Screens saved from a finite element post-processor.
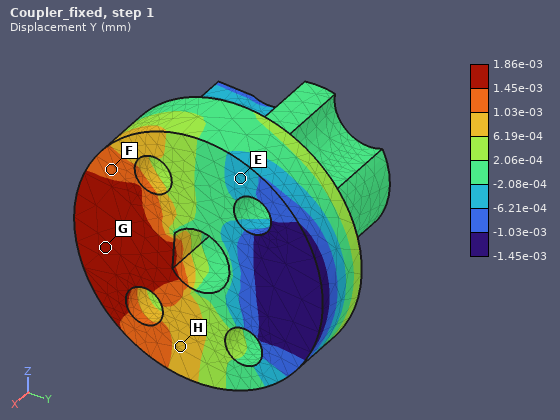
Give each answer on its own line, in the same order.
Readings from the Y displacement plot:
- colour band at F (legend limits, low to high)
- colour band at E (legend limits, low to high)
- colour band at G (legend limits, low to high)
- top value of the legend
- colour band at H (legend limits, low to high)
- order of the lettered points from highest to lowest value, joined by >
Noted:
1.03e-03 to 1.45e-03 mm
-6.21e-04 to -2.08e-04 mm
1.45e-03 to 1.86e-03 mm
1.86e-03 mm
6.19e-04 to 1.03e-03 mm
G > F > H > E
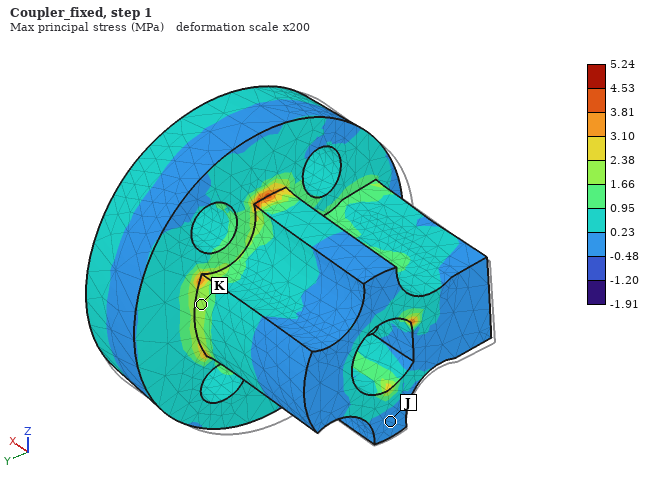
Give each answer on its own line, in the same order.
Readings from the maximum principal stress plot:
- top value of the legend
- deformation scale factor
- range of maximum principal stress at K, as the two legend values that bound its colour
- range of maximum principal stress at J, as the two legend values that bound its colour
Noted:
5.24 MPa
200
1.66 to 2.38 MPa
-0.48 to 0.23 MPa
